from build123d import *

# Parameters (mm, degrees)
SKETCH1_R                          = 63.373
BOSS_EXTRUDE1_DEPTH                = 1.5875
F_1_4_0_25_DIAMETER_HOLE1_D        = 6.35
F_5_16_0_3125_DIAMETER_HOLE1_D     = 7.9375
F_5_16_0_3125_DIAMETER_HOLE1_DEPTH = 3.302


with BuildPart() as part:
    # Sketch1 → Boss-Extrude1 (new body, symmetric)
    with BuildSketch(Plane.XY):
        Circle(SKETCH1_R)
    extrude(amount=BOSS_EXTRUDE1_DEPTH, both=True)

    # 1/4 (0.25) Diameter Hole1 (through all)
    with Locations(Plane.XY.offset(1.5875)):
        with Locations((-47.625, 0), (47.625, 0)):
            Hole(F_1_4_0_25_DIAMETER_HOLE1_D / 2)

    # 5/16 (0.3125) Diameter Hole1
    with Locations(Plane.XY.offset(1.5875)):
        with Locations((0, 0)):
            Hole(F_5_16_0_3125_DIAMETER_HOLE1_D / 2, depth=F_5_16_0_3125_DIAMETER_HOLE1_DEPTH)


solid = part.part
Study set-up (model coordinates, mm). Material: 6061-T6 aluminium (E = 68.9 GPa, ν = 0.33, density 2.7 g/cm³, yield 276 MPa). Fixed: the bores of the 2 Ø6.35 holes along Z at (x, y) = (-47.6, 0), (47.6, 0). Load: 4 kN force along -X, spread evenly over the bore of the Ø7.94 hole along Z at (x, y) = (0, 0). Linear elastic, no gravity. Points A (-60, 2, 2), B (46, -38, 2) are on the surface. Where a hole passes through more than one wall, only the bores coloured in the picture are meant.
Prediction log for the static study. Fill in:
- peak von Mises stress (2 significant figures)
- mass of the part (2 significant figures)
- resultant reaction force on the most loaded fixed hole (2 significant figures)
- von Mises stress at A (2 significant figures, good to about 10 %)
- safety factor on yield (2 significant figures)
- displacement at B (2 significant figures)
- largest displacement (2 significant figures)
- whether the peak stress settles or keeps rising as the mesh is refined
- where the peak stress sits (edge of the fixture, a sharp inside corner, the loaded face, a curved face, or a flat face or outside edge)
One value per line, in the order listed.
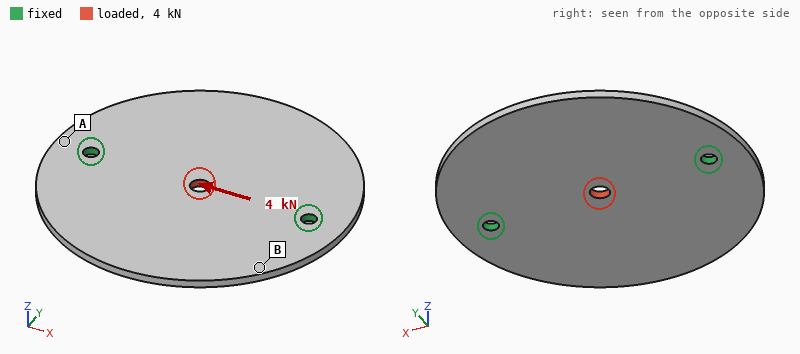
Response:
87 MPa
110 g
2.0 kN
10 MPa
3.2
7.7 µm
18 µm
settles
the loaded face
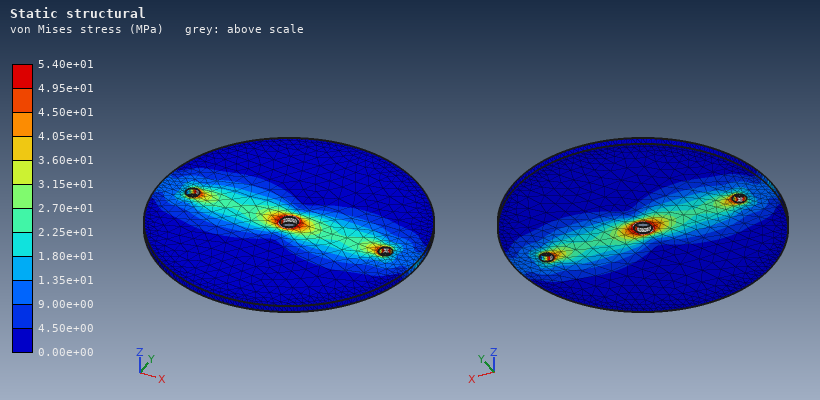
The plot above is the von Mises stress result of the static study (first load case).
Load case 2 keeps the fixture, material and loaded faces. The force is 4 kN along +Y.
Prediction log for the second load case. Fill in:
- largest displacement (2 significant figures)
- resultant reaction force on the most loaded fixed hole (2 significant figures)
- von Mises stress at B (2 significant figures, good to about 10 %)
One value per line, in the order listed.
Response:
24 µm
2.0 kN
7.5 MPa
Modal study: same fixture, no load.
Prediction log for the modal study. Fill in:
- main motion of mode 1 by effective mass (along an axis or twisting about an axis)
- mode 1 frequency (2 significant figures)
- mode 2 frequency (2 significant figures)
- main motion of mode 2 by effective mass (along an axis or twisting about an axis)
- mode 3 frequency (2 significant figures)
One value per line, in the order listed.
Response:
twisting about X
600 Hz
780 Hz
along Z
1700 Hz
